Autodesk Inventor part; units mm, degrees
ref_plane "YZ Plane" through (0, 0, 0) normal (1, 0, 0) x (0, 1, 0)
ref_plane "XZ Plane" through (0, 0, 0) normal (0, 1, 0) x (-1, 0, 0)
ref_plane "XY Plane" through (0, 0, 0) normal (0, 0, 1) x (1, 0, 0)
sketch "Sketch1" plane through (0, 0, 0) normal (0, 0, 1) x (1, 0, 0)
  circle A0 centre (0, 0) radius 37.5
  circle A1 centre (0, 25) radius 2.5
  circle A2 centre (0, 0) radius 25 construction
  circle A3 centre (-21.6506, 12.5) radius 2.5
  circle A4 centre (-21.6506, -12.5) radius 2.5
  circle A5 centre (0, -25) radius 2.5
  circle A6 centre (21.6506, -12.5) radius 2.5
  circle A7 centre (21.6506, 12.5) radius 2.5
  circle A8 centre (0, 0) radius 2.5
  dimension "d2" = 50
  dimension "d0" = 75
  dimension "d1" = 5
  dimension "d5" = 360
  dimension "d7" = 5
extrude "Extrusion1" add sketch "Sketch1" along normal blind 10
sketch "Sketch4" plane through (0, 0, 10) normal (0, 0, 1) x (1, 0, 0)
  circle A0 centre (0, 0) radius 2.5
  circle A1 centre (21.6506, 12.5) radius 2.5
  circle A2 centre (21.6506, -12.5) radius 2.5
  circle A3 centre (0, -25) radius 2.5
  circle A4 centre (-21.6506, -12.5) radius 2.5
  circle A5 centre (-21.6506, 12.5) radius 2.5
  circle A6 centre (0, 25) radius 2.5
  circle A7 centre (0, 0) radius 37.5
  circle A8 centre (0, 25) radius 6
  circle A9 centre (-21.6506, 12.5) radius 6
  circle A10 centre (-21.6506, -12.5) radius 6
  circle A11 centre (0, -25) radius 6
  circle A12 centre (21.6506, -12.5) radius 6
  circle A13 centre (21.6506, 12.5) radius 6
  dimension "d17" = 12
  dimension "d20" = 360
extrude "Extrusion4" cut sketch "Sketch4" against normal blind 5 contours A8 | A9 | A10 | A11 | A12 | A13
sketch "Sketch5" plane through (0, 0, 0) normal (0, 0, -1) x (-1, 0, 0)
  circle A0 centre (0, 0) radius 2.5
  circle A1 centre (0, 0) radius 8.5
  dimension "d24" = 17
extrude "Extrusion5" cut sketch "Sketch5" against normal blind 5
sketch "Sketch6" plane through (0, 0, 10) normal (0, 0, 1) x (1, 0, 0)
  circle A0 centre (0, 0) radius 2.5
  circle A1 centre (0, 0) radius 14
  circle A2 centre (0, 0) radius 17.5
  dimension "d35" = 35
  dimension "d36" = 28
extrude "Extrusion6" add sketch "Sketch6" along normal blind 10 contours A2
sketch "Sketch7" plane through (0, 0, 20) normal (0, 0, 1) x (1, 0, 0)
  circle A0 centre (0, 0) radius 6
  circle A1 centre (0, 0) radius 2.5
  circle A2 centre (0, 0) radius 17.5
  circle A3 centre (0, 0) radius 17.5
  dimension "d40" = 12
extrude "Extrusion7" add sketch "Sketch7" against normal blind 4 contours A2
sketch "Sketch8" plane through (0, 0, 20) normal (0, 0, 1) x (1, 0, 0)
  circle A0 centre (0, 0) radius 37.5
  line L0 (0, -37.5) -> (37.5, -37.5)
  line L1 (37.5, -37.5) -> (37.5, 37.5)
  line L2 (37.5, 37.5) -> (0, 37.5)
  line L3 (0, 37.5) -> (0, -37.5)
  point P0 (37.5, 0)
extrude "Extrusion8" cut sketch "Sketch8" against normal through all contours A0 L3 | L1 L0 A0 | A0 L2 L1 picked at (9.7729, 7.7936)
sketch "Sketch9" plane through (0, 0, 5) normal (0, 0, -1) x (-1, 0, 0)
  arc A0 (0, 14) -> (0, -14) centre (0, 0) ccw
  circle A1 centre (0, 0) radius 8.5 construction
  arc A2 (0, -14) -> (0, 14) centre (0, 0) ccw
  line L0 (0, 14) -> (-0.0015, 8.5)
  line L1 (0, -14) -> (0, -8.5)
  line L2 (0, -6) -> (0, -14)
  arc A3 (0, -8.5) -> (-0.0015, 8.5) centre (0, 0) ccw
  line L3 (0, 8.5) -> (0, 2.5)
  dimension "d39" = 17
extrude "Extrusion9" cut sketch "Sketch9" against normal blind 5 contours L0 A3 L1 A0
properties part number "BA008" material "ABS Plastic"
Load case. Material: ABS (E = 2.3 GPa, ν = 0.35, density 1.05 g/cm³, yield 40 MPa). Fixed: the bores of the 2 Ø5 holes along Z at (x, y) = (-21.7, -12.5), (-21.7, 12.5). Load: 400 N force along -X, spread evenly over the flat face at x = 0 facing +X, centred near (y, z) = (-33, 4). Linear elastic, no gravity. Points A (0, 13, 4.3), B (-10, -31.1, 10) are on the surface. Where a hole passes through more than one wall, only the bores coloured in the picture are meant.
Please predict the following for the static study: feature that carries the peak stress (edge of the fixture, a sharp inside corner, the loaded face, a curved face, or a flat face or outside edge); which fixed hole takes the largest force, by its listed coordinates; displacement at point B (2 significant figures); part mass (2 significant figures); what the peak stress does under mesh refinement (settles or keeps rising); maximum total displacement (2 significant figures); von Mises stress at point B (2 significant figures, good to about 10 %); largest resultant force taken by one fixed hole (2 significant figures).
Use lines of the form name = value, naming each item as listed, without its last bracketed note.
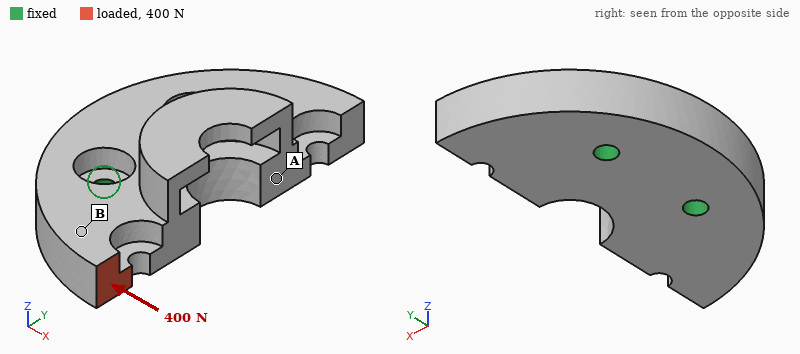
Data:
feature that carries the peak stress = edge of the fixture
which fixed hole takes the largest force, by its listed coordinates = (-21.7, -12.5)
displacement at point B = 0.18 mm
part mass = 23 g
what the peak stress does under mesh refinement = keeps rising
maximum total displacement = 0.30 mm
von Mises stress at point B = 4.2 MPa
largest resultant force taken by one fixed hole = 670 N
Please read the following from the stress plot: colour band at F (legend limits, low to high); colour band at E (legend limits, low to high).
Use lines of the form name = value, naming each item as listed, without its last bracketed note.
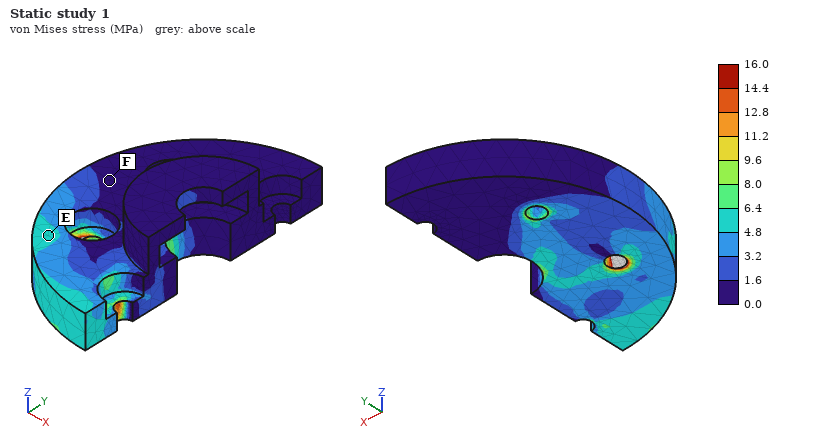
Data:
colour band at F = 0.0 to 1.6 MPa
colour band at E = 4.8 to 6.4 MPa
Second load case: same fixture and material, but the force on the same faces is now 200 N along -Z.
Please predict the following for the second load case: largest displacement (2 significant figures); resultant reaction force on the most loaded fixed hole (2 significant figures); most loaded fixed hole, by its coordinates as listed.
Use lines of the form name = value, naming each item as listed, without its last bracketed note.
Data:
largest displacement = 0.87 mm
resultant reaction force on the most loaded fixed hole = 340 N
most loaded fixed hole, by its coordinates as listed = (-21.7, -12.5)
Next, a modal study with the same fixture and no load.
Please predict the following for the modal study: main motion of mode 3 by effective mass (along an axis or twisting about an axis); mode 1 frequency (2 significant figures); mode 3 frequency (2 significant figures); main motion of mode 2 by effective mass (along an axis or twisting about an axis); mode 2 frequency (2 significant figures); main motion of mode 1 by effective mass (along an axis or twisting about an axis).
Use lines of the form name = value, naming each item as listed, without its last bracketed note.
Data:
main motion of mode 3 by effective mass = along Y
mode 1 frequency = 1700 Hz
mode 3 frequency = 3400 Hz
main motion of mode 2 by effective mass = twisting about X
mode 2 frequency = 2300 Hz
main motion of mode 1 by effective mass = along Z
